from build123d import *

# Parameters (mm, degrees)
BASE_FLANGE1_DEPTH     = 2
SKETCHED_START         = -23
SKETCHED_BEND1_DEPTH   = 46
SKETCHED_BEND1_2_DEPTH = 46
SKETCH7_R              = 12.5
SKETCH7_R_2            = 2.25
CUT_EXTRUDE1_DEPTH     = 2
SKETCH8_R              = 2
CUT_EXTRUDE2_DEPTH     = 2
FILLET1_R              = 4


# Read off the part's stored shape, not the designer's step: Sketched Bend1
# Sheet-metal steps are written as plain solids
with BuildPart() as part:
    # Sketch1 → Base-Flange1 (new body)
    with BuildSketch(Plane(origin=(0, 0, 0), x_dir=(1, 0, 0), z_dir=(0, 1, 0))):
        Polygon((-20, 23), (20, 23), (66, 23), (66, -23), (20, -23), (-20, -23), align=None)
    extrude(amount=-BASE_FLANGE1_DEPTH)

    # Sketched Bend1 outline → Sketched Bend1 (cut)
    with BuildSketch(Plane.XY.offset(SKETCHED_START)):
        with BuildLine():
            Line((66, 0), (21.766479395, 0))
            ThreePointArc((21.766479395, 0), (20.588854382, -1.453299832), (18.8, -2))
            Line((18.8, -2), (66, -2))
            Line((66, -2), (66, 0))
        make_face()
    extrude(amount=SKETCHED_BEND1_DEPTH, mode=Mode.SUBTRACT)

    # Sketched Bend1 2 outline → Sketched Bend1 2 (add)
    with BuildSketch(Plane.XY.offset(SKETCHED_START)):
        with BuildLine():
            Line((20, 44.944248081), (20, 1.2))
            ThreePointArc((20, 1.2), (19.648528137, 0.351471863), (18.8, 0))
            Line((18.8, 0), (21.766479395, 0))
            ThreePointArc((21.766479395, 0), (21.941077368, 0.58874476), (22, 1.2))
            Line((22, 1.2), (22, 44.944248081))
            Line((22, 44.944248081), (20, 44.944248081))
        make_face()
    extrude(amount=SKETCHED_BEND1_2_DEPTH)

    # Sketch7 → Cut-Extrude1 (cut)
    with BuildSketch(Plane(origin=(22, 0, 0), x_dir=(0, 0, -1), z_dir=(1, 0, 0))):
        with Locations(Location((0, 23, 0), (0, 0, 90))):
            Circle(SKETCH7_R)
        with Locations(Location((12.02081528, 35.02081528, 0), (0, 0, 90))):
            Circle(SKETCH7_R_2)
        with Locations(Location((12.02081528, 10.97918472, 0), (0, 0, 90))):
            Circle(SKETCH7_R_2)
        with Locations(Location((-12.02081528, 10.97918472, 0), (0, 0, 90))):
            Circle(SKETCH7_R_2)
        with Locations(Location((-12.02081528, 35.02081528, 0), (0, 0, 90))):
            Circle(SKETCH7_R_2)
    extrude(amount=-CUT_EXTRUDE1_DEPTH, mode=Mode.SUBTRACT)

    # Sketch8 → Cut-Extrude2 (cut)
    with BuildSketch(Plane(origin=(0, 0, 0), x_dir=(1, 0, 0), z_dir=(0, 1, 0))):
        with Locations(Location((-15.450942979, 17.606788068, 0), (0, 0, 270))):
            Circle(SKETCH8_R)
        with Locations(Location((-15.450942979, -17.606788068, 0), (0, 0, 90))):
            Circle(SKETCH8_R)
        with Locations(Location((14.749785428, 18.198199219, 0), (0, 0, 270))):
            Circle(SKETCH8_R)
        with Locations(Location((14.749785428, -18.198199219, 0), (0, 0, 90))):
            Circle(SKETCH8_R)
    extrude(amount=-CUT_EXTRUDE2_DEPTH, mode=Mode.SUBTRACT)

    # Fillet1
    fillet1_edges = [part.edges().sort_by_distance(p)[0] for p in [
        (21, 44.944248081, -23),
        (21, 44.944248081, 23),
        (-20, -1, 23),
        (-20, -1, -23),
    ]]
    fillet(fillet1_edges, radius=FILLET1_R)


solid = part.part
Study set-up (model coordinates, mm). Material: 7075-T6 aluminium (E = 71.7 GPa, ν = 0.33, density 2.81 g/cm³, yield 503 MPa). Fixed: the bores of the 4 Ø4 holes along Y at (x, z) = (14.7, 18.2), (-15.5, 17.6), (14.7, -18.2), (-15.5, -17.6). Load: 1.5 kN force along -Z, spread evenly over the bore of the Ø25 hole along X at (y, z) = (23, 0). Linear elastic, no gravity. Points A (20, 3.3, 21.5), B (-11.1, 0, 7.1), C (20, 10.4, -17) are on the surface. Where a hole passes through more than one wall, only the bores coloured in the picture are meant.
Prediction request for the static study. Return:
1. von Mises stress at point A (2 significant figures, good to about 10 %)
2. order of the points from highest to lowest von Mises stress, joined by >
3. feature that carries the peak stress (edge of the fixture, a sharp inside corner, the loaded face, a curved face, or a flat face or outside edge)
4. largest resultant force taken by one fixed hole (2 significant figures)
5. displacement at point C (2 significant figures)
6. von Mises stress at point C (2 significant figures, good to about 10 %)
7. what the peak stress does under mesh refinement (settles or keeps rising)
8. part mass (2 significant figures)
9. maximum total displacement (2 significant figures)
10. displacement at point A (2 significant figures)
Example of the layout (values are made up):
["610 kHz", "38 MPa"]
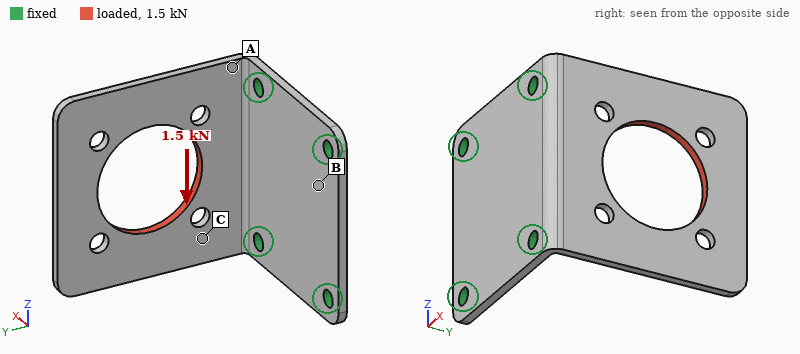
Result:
["150 MPa", "A > C > B", "edge of the fixture", "1.2 kN", "0.14 mm", "77 MPa", "keeps rising", "19 g", "0.37 mm", "0.098 mm"]
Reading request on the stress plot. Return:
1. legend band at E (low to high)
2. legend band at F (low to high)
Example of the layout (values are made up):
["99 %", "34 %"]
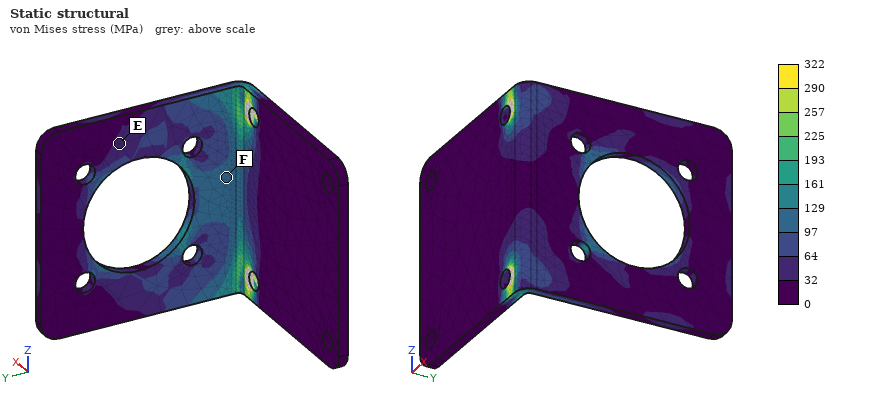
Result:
["32 to 64 MPa", "97 to 129 MPa"]
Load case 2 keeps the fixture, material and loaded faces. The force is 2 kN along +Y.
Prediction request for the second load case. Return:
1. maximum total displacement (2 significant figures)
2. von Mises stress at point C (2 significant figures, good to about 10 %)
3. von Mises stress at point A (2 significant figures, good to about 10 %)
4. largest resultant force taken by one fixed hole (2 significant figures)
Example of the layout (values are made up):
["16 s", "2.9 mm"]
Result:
["0.76 mm", "48 MPa", "79 MPa", "1.0 kN"]
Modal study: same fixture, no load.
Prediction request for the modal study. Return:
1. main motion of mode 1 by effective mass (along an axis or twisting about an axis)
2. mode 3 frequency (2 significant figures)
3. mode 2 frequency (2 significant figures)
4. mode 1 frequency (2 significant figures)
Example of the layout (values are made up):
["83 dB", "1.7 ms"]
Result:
["along X", "3800 Hz", "1500 Hz", "630 Hz"]
